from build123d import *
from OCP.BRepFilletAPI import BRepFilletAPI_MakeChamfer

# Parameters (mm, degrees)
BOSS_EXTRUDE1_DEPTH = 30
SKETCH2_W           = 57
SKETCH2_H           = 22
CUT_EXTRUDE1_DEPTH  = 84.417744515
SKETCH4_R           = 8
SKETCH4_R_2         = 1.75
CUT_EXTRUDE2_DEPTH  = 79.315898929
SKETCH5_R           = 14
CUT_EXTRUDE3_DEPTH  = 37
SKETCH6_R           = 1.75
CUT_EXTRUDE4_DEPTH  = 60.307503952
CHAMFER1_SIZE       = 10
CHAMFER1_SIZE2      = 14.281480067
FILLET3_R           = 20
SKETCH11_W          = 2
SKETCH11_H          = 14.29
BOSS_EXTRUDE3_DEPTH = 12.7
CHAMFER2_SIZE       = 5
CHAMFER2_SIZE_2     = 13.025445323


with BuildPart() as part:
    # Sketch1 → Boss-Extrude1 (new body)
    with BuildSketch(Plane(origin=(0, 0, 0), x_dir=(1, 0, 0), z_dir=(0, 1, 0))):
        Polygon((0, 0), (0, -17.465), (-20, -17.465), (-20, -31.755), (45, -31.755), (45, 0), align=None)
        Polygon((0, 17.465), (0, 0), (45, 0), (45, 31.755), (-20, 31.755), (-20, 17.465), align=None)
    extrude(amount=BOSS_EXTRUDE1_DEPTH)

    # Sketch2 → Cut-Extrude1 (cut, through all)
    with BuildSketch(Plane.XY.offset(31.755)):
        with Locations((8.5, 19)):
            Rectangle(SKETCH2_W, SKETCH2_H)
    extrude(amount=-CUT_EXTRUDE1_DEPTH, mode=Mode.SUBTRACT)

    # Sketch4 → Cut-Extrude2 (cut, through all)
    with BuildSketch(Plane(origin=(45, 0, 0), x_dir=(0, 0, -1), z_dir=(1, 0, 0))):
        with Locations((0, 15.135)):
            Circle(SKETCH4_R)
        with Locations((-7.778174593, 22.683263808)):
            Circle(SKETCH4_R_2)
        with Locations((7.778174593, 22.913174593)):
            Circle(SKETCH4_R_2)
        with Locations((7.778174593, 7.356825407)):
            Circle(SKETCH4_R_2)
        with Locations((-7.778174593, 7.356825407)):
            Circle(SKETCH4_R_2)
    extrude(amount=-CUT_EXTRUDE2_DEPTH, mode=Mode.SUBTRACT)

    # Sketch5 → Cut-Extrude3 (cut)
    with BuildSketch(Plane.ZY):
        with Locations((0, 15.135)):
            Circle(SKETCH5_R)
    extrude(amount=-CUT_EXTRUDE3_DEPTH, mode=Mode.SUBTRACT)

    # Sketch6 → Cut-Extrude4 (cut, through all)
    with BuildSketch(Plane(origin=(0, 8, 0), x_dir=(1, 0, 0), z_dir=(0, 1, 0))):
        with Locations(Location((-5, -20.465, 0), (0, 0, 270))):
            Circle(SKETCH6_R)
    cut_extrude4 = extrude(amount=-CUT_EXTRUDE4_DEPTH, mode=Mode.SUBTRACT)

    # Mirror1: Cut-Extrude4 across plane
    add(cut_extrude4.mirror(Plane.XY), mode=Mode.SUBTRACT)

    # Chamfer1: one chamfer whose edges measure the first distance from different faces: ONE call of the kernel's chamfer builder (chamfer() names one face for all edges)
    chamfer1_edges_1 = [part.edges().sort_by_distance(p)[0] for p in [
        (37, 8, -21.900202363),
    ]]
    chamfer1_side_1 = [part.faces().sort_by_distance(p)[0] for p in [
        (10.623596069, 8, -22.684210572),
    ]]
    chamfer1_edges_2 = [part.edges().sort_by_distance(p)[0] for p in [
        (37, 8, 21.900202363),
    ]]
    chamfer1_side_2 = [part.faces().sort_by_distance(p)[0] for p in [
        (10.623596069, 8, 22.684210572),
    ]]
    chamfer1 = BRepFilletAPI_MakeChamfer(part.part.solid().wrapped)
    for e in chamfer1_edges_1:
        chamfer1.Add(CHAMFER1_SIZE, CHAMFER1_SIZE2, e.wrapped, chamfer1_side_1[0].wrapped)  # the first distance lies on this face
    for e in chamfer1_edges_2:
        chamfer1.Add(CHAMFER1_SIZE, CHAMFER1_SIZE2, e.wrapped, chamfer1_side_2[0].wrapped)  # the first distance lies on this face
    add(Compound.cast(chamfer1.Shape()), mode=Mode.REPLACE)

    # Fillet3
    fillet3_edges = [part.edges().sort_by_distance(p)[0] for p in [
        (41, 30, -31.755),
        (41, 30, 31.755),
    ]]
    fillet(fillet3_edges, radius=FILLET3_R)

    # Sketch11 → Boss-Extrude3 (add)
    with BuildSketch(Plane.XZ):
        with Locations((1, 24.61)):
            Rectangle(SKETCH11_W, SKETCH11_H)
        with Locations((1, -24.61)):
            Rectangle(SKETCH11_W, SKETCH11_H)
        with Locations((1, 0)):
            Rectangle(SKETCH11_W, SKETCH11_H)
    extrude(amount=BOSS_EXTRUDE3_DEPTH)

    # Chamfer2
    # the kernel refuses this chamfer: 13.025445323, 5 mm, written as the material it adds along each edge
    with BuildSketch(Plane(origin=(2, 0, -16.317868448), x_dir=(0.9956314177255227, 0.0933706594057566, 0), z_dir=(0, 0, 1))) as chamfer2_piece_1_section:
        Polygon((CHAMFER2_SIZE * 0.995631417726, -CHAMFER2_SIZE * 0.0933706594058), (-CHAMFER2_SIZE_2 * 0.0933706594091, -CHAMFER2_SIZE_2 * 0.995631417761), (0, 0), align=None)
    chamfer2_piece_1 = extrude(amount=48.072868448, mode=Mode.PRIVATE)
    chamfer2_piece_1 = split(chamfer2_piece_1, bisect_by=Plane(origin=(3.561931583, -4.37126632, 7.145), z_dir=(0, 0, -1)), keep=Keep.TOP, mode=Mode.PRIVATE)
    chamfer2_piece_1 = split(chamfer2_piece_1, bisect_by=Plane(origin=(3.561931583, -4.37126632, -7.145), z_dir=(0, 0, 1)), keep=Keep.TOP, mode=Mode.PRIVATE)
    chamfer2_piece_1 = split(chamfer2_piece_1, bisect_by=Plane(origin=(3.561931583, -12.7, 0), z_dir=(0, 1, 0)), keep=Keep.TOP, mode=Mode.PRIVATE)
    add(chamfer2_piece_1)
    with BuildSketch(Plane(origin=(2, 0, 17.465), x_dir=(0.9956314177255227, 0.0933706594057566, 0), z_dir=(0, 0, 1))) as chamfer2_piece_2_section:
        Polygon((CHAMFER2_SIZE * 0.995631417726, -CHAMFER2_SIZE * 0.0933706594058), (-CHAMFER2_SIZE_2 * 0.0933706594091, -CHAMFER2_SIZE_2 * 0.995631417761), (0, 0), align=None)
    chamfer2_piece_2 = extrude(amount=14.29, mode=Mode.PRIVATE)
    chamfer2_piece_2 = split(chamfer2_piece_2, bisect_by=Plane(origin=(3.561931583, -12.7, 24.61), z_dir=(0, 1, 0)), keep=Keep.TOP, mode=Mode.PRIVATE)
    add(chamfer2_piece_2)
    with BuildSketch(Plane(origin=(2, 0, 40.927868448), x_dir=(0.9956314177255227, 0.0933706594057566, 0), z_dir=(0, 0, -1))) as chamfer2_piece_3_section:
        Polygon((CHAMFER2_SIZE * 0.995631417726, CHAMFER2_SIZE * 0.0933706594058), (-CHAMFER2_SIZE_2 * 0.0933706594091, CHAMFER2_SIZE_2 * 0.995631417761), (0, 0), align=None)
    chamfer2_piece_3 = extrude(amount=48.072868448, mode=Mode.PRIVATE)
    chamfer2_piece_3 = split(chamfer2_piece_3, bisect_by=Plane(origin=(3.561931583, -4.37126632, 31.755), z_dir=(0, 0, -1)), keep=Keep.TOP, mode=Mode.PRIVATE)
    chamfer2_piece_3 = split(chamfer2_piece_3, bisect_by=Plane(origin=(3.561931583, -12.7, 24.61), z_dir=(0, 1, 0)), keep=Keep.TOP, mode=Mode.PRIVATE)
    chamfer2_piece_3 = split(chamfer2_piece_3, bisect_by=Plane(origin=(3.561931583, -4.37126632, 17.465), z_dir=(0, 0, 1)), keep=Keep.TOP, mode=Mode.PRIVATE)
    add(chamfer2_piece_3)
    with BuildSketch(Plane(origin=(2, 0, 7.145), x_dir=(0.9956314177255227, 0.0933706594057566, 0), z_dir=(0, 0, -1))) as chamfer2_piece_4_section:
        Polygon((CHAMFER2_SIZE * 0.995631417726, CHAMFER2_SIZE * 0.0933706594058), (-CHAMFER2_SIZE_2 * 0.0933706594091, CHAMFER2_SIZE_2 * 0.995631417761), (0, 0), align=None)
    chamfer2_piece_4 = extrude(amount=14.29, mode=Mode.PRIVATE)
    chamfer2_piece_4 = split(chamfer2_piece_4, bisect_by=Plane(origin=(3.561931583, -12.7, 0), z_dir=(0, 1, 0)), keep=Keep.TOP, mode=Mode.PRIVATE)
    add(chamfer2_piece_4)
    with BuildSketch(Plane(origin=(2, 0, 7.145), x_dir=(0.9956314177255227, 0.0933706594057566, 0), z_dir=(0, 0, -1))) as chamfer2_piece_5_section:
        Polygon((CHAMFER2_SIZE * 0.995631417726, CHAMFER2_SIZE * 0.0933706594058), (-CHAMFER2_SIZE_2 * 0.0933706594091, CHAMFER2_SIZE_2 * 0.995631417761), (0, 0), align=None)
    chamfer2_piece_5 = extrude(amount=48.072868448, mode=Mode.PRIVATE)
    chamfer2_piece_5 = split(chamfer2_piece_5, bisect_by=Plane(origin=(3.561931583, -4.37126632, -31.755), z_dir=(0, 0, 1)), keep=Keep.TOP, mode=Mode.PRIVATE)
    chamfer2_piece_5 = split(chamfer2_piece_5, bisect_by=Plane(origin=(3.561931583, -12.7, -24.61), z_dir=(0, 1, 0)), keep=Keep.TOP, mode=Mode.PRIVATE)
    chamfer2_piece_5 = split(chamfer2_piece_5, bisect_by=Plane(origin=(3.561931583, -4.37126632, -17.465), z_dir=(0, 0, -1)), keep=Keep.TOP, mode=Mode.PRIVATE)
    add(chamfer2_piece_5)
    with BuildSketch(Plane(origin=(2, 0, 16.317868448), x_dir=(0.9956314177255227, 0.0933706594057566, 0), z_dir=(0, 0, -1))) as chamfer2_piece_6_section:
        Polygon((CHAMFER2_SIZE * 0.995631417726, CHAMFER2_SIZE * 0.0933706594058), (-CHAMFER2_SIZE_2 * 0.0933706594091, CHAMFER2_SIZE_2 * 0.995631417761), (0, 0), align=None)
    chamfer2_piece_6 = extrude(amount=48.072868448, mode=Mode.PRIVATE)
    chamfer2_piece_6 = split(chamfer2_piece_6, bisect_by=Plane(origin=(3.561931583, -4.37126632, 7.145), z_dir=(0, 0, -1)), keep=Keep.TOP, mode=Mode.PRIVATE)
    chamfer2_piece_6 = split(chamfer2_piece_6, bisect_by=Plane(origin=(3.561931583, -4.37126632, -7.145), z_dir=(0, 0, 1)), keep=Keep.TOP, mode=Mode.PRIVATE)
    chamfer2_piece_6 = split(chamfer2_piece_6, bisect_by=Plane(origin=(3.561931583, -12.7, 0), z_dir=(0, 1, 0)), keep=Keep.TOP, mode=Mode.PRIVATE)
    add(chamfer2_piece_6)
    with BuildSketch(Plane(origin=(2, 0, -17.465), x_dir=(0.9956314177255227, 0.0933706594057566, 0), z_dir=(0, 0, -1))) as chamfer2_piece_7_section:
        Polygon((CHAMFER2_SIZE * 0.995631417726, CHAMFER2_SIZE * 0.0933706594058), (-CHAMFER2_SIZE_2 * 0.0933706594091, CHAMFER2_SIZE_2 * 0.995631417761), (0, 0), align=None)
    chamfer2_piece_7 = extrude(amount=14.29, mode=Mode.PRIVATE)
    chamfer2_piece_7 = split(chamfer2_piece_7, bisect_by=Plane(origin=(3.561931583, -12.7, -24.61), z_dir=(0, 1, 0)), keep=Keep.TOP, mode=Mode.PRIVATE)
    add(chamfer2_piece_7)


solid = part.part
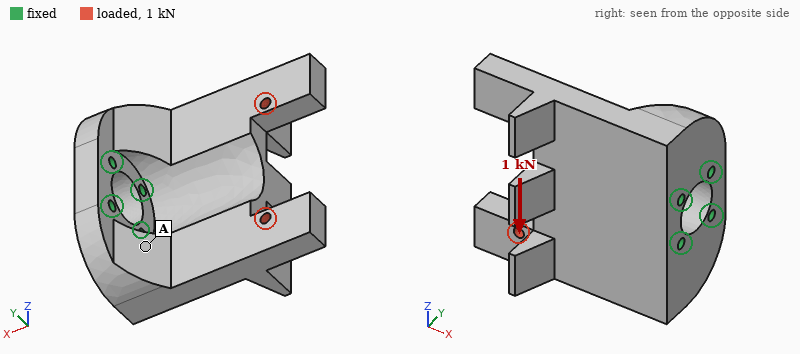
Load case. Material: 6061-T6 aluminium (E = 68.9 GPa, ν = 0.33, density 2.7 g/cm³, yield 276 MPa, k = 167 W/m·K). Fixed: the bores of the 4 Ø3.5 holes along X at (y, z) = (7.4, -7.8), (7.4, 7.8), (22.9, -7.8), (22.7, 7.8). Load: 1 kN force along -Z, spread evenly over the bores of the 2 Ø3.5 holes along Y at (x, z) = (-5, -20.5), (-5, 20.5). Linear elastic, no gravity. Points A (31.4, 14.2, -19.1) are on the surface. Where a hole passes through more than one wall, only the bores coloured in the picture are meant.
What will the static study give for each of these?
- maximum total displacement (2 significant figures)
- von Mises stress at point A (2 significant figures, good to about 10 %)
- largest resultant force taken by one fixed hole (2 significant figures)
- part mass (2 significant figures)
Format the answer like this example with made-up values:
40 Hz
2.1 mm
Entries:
0.11 mm
12 MPa
1.5 kN
97 g
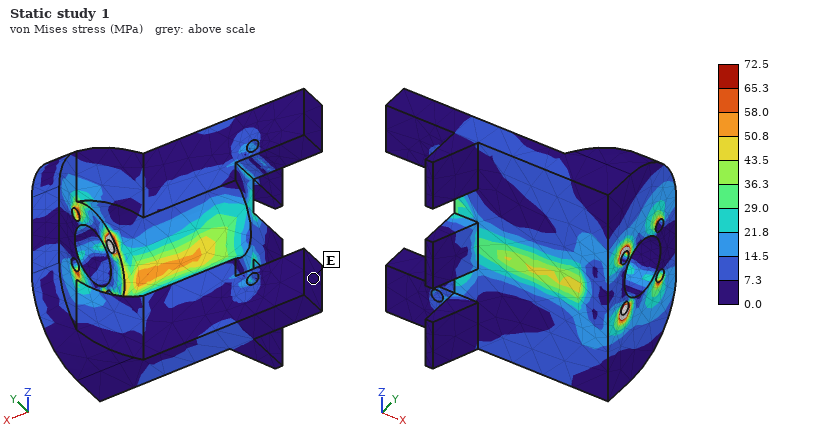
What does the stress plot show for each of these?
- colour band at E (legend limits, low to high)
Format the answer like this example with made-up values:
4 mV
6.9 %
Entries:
0.0 to 7.3 MPa
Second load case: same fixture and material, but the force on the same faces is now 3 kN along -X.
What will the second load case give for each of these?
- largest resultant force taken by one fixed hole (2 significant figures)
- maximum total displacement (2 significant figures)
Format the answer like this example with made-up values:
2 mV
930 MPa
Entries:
1.6 kN
22 µm
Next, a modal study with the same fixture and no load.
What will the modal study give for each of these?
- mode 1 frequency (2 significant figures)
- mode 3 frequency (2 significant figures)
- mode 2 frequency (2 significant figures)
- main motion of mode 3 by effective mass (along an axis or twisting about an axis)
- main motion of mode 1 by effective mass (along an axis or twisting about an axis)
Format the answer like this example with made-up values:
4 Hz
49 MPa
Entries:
2300 Hz
3700 Hz
2500 Hz
along Z
along Y
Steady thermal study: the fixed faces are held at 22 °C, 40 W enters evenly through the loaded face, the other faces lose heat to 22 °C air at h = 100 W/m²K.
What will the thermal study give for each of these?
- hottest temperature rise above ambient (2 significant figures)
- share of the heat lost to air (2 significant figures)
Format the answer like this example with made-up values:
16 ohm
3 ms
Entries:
30 K
35 %
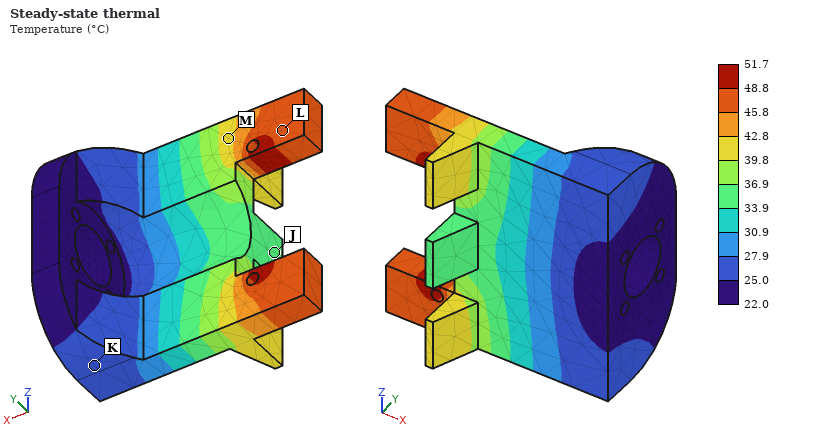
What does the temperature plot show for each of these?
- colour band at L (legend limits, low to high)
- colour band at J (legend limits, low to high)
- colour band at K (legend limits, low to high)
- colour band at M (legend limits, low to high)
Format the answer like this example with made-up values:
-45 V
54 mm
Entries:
45.8 to 48.8 °C
33.9 to 36.9 °C
25.0 to 27.9 °C
39.8 to 42.8 °C
